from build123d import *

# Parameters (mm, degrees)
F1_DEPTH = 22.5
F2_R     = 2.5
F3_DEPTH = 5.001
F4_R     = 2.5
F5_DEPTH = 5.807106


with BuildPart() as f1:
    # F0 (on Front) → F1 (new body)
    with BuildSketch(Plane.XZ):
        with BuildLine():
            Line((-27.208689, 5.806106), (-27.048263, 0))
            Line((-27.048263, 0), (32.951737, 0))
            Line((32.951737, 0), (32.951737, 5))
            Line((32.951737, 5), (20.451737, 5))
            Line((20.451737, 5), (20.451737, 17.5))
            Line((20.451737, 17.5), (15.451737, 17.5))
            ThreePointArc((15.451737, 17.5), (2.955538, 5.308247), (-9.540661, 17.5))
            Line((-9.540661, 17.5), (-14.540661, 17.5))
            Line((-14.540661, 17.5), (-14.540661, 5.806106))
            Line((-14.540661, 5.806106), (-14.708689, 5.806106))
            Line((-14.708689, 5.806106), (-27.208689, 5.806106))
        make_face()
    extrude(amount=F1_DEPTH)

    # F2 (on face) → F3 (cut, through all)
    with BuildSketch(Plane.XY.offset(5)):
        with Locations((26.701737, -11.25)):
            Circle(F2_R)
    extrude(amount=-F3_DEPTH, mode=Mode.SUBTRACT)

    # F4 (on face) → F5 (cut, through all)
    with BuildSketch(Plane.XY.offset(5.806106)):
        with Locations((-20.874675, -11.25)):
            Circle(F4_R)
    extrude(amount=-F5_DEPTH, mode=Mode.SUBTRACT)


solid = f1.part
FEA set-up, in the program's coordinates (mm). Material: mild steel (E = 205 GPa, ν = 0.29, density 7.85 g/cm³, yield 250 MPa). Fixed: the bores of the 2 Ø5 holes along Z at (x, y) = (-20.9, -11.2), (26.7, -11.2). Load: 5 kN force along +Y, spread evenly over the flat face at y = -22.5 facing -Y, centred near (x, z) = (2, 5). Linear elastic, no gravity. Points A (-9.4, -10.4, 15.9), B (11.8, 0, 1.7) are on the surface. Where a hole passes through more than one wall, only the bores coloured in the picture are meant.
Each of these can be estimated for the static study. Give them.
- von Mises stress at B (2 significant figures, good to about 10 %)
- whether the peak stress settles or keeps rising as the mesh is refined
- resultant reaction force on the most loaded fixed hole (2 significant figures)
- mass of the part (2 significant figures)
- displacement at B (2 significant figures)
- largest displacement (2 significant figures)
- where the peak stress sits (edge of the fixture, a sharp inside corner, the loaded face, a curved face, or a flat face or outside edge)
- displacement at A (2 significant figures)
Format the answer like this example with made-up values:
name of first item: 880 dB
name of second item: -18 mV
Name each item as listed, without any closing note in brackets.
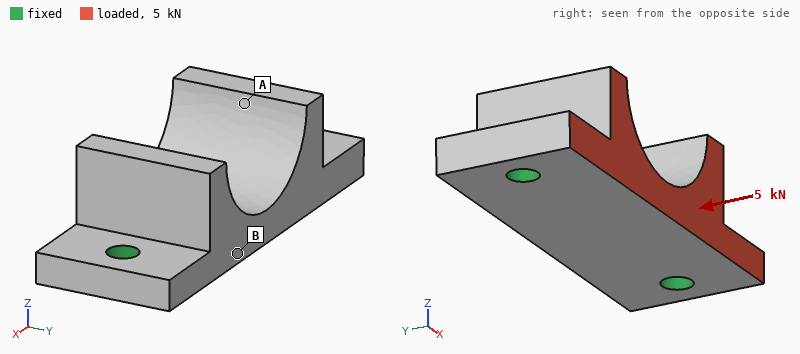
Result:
von Mises stress at B: 32 MPa
whether the peak stress settles or keeps rising as the mesh is refined: keeps rising
resultant reaction force on the most loaded fixed hole: 2.6 kN
mass of the part: 88 g
displacement at B: 7.6 µm
largest displacement: 15 µm
where the peak stress sits: edge of the fixture
displacement at A: 10 µm
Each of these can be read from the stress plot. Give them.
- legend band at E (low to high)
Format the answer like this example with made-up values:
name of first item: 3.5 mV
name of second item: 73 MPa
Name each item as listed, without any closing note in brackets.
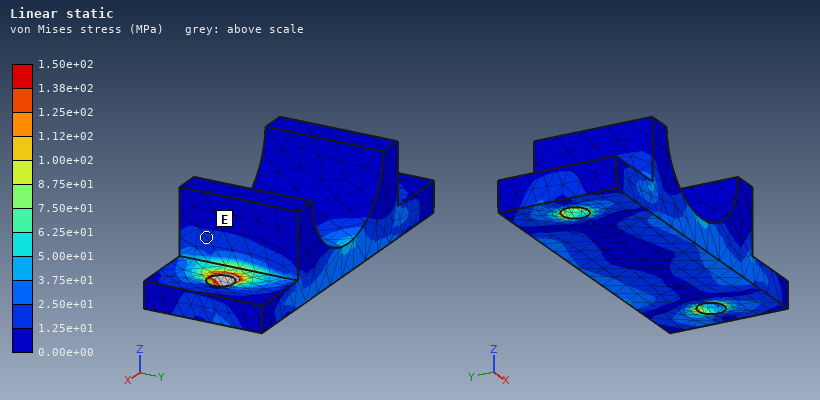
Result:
legend band at E: 1.25e+01 to 2.50e+01 MPa
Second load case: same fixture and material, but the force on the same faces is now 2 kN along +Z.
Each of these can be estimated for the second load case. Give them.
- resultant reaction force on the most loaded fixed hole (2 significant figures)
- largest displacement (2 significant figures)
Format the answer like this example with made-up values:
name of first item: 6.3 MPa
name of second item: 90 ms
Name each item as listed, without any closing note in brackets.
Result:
resultant reaction force on the most loaded fixed hole: 1.1 kN
largest displacement: 21 µm
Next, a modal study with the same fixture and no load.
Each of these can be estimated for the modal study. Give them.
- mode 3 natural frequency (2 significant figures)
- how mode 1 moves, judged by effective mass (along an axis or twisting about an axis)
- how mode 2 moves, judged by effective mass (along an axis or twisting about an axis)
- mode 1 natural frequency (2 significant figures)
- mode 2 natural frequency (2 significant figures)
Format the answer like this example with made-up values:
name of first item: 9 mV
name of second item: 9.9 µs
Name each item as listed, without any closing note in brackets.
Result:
mode 3 natural frequency: 17 kHz
how mode 1 moves, judged by effective mass: along Z
how mode 2 moves, judged by effective mass: along Y
mode 1 natural frequency: 9200 Hz
mode 2 natural frequency: 10 kHz
